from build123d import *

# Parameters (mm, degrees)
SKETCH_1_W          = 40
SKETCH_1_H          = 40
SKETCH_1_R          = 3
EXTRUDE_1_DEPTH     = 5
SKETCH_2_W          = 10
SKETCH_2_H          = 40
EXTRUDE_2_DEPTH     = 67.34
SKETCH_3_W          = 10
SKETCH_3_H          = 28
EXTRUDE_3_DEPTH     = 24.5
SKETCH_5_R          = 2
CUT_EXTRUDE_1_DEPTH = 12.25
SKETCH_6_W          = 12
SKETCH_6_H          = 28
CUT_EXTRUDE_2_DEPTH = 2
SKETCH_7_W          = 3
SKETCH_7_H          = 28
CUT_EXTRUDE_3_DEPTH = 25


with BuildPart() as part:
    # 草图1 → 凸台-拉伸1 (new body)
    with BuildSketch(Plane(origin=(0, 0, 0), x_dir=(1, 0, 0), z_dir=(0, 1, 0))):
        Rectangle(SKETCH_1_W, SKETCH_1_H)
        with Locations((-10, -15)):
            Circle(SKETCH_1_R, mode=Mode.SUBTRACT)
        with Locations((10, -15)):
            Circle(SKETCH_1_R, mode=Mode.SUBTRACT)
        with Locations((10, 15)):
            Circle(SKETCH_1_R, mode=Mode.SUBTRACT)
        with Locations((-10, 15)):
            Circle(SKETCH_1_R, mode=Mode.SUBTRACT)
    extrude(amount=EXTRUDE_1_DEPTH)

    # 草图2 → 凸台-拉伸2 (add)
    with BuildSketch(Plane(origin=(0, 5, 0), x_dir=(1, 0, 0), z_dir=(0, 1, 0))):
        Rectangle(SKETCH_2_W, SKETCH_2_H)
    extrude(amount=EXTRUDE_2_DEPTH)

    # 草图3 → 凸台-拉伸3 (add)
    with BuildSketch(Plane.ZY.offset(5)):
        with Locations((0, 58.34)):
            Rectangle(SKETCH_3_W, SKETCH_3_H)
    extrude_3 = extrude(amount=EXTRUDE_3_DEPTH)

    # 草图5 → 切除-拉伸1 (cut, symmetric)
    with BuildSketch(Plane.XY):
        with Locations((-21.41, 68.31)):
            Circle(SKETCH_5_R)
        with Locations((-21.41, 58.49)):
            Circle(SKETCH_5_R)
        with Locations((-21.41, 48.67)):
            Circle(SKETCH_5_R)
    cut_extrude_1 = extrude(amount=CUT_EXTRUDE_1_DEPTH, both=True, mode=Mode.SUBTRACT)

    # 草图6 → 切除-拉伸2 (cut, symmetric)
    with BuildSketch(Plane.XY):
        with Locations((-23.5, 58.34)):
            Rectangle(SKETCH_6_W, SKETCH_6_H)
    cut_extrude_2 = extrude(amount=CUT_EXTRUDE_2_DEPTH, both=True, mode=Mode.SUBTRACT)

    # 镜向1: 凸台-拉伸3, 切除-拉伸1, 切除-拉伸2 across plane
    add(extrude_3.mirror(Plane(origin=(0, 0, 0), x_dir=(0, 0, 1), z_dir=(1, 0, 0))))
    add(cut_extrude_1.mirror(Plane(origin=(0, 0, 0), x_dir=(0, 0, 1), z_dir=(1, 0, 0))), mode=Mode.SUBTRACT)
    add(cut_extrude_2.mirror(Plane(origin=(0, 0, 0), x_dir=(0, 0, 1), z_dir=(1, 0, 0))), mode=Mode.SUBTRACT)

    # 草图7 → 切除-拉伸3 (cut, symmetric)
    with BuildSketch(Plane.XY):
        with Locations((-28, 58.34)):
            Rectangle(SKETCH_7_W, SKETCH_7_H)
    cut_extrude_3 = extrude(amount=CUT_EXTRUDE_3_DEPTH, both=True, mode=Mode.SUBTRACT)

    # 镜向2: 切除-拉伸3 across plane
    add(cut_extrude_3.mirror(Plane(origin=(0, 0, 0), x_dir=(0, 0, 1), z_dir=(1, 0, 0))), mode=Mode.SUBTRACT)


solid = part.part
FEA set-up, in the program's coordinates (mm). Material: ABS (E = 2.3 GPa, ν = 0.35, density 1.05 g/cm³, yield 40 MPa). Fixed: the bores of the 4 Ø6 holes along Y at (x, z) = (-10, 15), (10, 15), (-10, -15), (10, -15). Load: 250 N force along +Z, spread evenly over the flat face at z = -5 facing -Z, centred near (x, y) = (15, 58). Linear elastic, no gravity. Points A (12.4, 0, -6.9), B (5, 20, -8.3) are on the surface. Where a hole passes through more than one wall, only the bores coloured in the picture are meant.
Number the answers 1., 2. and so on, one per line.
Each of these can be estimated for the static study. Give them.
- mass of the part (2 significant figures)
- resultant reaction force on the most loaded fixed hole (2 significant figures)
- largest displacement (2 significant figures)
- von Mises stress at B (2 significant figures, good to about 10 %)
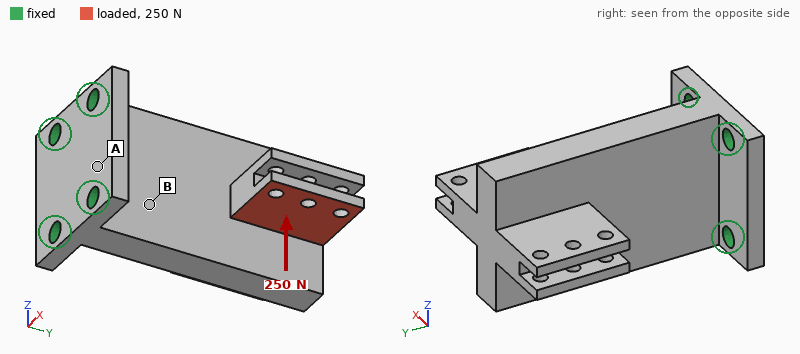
1. 46 g
2. 330 N
3. 0.99 mm
4. 6.1 MPa
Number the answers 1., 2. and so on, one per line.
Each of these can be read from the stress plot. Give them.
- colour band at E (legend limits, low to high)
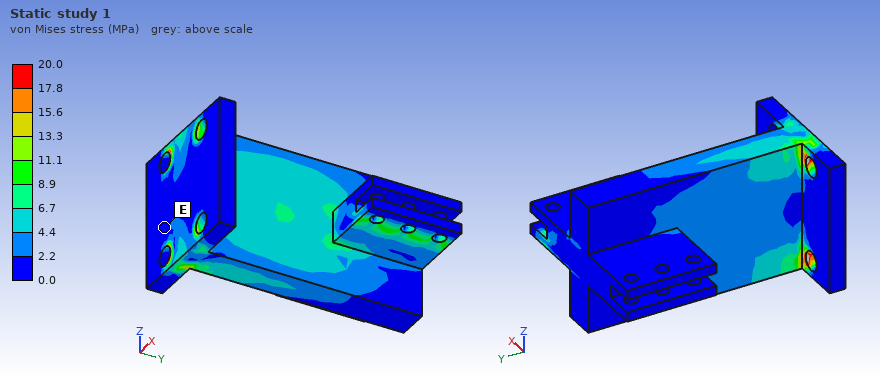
1. 0.0 to 2.2 MPa
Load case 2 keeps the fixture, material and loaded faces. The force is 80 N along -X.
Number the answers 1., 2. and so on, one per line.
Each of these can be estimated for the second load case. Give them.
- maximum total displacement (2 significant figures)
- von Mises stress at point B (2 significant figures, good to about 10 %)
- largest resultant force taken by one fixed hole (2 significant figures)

1. 1.1 mm
2. 4.4 MPa
3. 160 N
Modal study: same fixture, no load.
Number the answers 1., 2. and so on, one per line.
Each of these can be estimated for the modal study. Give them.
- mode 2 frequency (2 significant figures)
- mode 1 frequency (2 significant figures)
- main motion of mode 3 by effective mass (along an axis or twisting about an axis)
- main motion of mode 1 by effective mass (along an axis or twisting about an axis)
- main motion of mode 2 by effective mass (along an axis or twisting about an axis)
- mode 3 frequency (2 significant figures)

1. 960 Hz
2. 330 Hz
3. twisting about Y
4. along X
5. along Z
6. 1100 Hz
